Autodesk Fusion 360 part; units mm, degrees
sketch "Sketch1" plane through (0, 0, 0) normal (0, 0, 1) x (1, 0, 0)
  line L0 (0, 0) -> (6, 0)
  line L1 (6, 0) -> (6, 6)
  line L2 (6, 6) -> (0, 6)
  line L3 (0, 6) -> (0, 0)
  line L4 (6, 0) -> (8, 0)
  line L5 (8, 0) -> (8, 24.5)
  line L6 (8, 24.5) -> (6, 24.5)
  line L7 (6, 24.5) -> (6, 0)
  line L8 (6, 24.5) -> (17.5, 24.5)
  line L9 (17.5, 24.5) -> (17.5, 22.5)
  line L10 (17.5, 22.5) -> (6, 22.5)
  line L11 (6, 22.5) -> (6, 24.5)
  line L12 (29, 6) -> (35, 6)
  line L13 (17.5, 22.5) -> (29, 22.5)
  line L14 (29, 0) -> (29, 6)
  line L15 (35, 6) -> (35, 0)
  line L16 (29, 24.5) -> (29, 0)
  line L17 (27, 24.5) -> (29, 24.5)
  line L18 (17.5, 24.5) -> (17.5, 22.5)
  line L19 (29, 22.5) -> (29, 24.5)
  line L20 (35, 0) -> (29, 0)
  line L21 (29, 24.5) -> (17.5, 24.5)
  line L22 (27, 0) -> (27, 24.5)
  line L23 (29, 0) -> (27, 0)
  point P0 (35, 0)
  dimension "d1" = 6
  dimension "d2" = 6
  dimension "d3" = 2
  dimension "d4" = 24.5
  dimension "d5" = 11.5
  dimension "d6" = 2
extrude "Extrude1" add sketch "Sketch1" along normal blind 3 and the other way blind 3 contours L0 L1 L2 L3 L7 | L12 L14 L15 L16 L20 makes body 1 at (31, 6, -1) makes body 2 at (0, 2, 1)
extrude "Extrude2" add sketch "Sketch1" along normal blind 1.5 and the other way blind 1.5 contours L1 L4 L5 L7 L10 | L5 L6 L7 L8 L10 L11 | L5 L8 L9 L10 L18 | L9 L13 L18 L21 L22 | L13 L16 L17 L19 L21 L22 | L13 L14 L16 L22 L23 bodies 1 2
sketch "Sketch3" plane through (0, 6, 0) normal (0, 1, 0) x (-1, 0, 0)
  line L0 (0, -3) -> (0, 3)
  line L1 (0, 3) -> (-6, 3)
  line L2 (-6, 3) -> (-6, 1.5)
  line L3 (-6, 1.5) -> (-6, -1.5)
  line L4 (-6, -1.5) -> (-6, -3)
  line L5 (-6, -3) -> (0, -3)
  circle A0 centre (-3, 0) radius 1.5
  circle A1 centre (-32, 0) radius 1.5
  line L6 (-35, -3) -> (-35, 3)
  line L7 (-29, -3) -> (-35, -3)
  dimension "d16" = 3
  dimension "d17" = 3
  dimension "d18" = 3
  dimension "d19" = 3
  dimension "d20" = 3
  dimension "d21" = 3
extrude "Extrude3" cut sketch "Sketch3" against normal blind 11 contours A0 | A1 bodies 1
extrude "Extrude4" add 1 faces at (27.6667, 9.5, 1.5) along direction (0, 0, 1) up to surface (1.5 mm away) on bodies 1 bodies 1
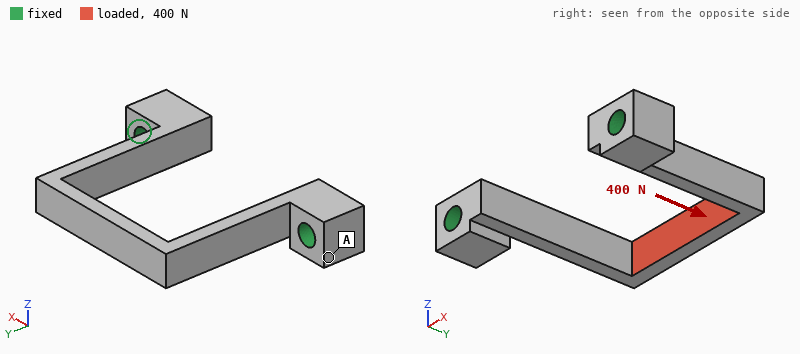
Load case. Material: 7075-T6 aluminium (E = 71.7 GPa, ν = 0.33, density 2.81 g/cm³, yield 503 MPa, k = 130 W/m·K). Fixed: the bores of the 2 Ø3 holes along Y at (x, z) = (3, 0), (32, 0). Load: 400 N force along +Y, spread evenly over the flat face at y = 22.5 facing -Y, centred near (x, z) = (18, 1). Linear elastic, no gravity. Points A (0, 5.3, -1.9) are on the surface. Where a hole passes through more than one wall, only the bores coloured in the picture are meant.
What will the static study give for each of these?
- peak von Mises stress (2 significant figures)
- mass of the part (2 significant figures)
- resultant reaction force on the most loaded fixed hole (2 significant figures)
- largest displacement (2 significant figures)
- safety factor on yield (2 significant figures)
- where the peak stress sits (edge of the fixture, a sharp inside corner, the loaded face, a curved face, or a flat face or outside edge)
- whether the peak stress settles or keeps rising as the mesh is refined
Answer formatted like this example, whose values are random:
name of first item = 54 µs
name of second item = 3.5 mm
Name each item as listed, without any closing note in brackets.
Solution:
peak von Mises stress = 200 MPa
mass of the part = 2.7 g
resultant reaction force on the most loaded fixed hole = 210 N
largest displacement = 0.11 mm
safety factor on yield = 2.5
where the peak stress sits = a flat face or outside edge
whether the peak stress settles or keeps rising as the mesh is refined = settles
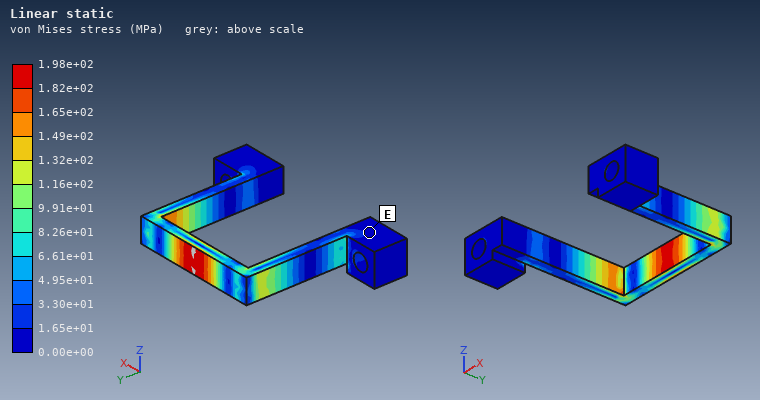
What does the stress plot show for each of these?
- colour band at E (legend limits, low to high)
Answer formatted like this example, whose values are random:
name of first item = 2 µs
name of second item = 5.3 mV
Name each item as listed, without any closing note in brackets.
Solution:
colour band at E = 0.00e+00 to 1.65e+01 MPa
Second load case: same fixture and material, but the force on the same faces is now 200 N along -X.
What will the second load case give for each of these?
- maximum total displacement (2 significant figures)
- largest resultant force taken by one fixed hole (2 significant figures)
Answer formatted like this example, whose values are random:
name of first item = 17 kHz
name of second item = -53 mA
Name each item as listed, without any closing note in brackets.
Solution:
maximum total displacement = 0.36 mm
largest resultant force taken by one fixed hole = 120 N
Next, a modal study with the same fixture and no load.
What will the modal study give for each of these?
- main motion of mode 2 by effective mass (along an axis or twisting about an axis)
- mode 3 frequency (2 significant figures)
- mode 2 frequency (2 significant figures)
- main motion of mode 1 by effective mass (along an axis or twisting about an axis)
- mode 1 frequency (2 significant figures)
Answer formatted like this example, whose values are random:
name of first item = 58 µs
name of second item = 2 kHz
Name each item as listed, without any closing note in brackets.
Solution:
main motion of mode 2 by effective mass = along Z
mode 3 frequency = 8200 Hz
mode 2 frequency = 5000 Hz
main motion of mode 1 by effective mass = along X
mode 1 frequency = 4200 Hz
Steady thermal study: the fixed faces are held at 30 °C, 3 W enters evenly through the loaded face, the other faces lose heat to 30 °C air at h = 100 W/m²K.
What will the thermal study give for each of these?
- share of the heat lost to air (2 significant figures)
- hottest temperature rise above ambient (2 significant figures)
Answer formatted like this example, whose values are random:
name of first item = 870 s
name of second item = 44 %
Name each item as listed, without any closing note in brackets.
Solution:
share of the heat lost to air = 29 %
hottest temperature rise above ambient = 25 K
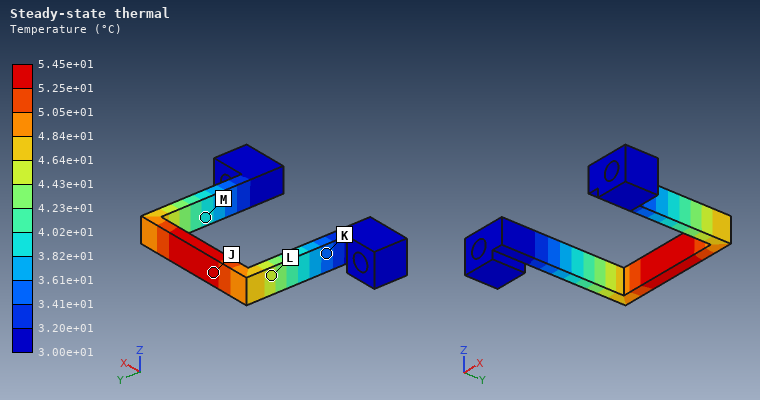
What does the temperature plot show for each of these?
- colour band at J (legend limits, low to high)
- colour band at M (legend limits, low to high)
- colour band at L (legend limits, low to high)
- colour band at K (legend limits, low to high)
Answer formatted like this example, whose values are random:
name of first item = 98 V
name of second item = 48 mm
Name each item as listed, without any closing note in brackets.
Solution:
colour band at J = 5.25e+01 to 5.45e+01 °C
colour band at M = 3.82e+01 to 4.02e+01 °C
colour band at L = 4.43e+01 to 4.64e+01 °C
colour band at K = 3.41e+01 to 3.61e+01 °C
